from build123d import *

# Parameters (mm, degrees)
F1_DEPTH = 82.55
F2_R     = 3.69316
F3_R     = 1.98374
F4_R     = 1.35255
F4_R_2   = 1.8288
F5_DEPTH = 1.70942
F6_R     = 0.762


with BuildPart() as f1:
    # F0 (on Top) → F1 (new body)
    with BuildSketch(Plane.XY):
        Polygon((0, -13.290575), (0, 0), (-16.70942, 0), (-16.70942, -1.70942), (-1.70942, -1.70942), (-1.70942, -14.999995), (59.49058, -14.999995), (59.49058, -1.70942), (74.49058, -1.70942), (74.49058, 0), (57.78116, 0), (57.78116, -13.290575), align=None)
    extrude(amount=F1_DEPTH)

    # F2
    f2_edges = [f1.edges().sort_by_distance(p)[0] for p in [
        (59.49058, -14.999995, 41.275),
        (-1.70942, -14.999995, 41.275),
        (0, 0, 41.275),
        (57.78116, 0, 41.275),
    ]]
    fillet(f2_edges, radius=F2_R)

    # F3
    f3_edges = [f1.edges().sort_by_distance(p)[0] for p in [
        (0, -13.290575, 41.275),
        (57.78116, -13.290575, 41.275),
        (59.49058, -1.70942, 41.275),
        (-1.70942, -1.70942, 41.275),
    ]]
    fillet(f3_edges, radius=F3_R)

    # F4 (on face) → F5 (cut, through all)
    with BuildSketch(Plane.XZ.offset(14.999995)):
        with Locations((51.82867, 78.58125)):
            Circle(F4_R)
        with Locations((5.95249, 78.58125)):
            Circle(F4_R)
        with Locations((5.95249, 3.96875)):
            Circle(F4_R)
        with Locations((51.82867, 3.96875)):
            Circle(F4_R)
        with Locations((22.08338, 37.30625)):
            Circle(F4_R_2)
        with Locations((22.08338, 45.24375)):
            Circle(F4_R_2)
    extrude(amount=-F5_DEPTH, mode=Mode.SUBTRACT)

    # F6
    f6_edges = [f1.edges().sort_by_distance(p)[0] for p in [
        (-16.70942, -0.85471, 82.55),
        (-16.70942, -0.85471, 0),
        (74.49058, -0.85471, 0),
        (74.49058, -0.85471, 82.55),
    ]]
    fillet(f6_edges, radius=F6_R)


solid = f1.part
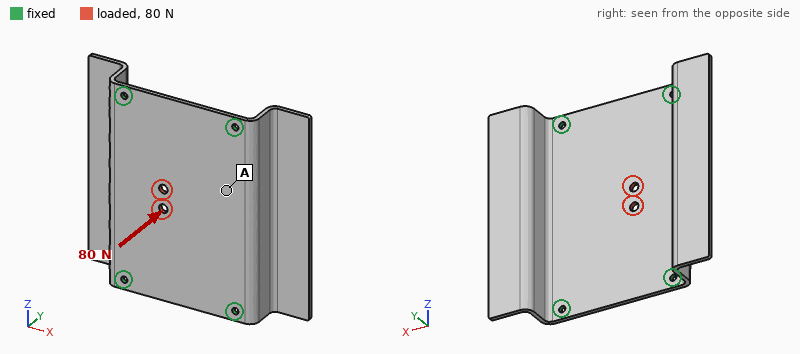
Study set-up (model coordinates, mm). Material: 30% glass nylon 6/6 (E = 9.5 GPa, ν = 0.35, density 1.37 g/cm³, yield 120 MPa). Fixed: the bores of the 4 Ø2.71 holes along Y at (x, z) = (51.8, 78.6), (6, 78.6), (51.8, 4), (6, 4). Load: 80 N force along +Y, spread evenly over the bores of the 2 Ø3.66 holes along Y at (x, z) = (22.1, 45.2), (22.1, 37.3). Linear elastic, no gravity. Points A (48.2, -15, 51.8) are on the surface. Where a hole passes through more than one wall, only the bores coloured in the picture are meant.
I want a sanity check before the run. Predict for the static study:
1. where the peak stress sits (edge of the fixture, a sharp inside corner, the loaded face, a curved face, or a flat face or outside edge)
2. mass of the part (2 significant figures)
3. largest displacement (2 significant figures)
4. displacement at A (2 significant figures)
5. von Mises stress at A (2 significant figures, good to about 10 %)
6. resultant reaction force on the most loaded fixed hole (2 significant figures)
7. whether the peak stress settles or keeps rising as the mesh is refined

a sharp inside corner
22 g
0.64 mm
0.16 mm
5.7 MPa
37 N
keeps rising
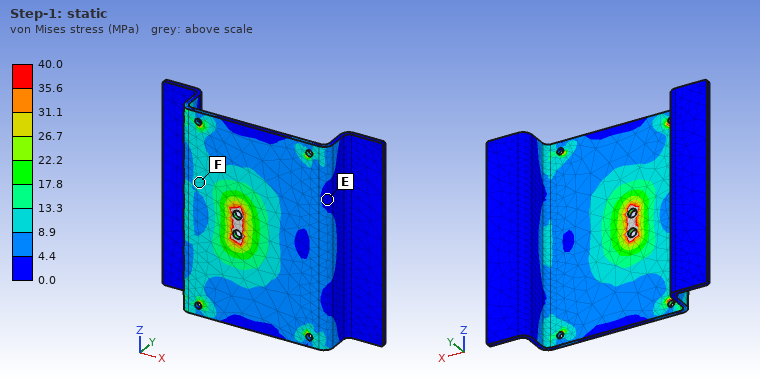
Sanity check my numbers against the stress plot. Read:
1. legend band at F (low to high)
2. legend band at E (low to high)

8.9 to 13.3 MPa
0.0 to 4.4 MPa
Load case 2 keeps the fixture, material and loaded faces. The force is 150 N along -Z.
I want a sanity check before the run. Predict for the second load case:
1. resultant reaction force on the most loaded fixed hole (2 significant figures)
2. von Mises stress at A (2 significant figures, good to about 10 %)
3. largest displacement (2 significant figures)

45 N
0.44 MPa
10 µm
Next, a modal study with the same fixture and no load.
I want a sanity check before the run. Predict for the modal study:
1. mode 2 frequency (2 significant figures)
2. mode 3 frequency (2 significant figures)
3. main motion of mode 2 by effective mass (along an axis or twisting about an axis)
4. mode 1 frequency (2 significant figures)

740 Hz
1100 Hz
along X
660 Hz
